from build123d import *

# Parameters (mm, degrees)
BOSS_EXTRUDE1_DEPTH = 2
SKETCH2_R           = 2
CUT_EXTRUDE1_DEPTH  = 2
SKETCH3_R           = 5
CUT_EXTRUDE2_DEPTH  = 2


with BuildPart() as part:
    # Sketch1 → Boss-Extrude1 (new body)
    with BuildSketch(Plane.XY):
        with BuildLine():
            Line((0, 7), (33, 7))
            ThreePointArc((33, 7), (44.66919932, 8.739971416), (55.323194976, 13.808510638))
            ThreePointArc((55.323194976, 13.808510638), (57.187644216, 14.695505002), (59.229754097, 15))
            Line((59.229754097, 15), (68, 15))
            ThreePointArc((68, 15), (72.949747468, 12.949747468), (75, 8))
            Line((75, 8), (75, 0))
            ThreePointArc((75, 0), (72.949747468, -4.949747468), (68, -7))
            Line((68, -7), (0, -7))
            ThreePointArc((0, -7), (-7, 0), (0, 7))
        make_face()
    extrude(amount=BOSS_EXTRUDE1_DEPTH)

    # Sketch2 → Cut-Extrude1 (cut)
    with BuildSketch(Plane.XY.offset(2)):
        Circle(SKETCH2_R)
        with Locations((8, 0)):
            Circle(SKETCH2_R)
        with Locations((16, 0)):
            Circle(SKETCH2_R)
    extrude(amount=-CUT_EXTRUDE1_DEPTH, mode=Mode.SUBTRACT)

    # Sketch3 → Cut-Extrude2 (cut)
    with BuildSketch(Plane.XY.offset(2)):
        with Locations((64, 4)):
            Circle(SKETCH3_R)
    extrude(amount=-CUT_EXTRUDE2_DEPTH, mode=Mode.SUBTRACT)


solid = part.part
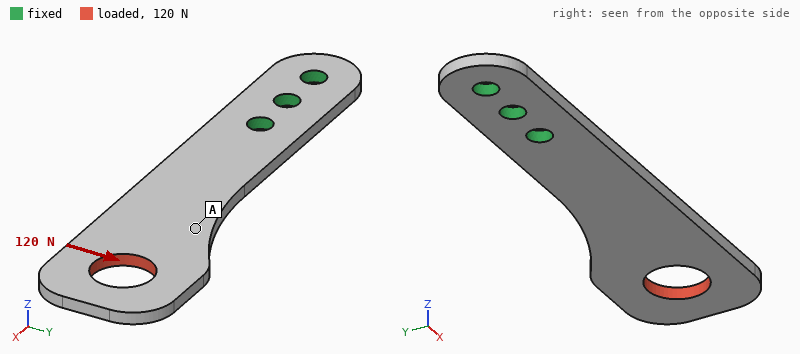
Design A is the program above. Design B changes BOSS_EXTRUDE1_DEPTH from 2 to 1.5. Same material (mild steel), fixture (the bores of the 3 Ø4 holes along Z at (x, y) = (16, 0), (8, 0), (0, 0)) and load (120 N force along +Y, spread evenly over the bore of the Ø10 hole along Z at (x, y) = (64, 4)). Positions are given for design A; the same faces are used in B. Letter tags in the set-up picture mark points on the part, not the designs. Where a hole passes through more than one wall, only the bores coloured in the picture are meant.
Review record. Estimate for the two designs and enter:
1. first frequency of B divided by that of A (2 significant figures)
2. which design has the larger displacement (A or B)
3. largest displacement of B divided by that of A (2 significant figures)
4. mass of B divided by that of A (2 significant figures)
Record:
0.75
B
1.3
0.75
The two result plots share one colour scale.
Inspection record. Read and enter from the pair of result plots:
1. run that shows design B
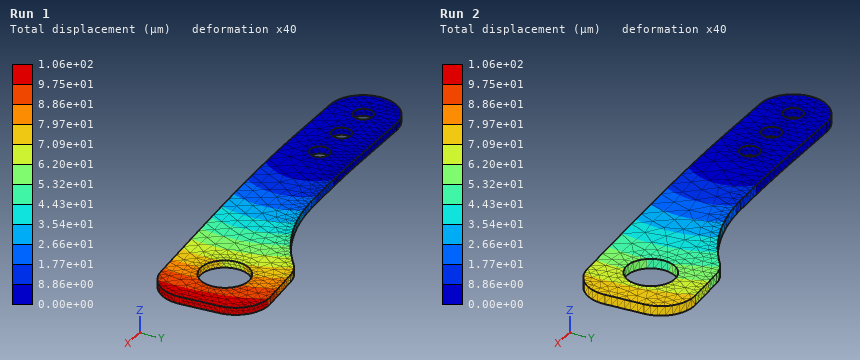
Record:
Run 1
